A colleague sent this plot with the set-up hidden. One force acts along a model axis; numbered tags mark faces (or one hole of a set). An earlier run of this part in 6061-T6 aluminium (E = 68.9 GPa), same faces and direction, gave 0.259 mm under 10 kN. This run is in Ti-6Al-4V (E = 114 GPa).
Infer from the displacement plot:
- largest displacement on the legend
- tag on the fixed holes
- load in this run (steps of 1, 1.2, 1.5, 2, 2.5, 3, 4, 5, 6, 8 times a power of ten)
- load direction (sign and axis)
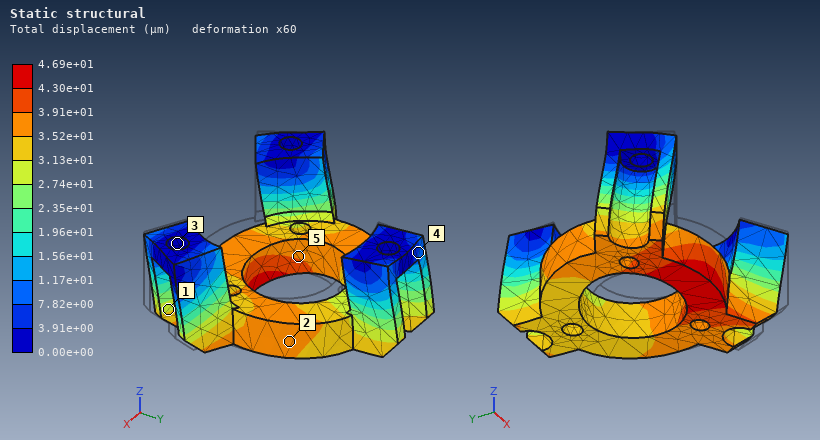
4.69e+01 µm
3
3 kN
+Y
